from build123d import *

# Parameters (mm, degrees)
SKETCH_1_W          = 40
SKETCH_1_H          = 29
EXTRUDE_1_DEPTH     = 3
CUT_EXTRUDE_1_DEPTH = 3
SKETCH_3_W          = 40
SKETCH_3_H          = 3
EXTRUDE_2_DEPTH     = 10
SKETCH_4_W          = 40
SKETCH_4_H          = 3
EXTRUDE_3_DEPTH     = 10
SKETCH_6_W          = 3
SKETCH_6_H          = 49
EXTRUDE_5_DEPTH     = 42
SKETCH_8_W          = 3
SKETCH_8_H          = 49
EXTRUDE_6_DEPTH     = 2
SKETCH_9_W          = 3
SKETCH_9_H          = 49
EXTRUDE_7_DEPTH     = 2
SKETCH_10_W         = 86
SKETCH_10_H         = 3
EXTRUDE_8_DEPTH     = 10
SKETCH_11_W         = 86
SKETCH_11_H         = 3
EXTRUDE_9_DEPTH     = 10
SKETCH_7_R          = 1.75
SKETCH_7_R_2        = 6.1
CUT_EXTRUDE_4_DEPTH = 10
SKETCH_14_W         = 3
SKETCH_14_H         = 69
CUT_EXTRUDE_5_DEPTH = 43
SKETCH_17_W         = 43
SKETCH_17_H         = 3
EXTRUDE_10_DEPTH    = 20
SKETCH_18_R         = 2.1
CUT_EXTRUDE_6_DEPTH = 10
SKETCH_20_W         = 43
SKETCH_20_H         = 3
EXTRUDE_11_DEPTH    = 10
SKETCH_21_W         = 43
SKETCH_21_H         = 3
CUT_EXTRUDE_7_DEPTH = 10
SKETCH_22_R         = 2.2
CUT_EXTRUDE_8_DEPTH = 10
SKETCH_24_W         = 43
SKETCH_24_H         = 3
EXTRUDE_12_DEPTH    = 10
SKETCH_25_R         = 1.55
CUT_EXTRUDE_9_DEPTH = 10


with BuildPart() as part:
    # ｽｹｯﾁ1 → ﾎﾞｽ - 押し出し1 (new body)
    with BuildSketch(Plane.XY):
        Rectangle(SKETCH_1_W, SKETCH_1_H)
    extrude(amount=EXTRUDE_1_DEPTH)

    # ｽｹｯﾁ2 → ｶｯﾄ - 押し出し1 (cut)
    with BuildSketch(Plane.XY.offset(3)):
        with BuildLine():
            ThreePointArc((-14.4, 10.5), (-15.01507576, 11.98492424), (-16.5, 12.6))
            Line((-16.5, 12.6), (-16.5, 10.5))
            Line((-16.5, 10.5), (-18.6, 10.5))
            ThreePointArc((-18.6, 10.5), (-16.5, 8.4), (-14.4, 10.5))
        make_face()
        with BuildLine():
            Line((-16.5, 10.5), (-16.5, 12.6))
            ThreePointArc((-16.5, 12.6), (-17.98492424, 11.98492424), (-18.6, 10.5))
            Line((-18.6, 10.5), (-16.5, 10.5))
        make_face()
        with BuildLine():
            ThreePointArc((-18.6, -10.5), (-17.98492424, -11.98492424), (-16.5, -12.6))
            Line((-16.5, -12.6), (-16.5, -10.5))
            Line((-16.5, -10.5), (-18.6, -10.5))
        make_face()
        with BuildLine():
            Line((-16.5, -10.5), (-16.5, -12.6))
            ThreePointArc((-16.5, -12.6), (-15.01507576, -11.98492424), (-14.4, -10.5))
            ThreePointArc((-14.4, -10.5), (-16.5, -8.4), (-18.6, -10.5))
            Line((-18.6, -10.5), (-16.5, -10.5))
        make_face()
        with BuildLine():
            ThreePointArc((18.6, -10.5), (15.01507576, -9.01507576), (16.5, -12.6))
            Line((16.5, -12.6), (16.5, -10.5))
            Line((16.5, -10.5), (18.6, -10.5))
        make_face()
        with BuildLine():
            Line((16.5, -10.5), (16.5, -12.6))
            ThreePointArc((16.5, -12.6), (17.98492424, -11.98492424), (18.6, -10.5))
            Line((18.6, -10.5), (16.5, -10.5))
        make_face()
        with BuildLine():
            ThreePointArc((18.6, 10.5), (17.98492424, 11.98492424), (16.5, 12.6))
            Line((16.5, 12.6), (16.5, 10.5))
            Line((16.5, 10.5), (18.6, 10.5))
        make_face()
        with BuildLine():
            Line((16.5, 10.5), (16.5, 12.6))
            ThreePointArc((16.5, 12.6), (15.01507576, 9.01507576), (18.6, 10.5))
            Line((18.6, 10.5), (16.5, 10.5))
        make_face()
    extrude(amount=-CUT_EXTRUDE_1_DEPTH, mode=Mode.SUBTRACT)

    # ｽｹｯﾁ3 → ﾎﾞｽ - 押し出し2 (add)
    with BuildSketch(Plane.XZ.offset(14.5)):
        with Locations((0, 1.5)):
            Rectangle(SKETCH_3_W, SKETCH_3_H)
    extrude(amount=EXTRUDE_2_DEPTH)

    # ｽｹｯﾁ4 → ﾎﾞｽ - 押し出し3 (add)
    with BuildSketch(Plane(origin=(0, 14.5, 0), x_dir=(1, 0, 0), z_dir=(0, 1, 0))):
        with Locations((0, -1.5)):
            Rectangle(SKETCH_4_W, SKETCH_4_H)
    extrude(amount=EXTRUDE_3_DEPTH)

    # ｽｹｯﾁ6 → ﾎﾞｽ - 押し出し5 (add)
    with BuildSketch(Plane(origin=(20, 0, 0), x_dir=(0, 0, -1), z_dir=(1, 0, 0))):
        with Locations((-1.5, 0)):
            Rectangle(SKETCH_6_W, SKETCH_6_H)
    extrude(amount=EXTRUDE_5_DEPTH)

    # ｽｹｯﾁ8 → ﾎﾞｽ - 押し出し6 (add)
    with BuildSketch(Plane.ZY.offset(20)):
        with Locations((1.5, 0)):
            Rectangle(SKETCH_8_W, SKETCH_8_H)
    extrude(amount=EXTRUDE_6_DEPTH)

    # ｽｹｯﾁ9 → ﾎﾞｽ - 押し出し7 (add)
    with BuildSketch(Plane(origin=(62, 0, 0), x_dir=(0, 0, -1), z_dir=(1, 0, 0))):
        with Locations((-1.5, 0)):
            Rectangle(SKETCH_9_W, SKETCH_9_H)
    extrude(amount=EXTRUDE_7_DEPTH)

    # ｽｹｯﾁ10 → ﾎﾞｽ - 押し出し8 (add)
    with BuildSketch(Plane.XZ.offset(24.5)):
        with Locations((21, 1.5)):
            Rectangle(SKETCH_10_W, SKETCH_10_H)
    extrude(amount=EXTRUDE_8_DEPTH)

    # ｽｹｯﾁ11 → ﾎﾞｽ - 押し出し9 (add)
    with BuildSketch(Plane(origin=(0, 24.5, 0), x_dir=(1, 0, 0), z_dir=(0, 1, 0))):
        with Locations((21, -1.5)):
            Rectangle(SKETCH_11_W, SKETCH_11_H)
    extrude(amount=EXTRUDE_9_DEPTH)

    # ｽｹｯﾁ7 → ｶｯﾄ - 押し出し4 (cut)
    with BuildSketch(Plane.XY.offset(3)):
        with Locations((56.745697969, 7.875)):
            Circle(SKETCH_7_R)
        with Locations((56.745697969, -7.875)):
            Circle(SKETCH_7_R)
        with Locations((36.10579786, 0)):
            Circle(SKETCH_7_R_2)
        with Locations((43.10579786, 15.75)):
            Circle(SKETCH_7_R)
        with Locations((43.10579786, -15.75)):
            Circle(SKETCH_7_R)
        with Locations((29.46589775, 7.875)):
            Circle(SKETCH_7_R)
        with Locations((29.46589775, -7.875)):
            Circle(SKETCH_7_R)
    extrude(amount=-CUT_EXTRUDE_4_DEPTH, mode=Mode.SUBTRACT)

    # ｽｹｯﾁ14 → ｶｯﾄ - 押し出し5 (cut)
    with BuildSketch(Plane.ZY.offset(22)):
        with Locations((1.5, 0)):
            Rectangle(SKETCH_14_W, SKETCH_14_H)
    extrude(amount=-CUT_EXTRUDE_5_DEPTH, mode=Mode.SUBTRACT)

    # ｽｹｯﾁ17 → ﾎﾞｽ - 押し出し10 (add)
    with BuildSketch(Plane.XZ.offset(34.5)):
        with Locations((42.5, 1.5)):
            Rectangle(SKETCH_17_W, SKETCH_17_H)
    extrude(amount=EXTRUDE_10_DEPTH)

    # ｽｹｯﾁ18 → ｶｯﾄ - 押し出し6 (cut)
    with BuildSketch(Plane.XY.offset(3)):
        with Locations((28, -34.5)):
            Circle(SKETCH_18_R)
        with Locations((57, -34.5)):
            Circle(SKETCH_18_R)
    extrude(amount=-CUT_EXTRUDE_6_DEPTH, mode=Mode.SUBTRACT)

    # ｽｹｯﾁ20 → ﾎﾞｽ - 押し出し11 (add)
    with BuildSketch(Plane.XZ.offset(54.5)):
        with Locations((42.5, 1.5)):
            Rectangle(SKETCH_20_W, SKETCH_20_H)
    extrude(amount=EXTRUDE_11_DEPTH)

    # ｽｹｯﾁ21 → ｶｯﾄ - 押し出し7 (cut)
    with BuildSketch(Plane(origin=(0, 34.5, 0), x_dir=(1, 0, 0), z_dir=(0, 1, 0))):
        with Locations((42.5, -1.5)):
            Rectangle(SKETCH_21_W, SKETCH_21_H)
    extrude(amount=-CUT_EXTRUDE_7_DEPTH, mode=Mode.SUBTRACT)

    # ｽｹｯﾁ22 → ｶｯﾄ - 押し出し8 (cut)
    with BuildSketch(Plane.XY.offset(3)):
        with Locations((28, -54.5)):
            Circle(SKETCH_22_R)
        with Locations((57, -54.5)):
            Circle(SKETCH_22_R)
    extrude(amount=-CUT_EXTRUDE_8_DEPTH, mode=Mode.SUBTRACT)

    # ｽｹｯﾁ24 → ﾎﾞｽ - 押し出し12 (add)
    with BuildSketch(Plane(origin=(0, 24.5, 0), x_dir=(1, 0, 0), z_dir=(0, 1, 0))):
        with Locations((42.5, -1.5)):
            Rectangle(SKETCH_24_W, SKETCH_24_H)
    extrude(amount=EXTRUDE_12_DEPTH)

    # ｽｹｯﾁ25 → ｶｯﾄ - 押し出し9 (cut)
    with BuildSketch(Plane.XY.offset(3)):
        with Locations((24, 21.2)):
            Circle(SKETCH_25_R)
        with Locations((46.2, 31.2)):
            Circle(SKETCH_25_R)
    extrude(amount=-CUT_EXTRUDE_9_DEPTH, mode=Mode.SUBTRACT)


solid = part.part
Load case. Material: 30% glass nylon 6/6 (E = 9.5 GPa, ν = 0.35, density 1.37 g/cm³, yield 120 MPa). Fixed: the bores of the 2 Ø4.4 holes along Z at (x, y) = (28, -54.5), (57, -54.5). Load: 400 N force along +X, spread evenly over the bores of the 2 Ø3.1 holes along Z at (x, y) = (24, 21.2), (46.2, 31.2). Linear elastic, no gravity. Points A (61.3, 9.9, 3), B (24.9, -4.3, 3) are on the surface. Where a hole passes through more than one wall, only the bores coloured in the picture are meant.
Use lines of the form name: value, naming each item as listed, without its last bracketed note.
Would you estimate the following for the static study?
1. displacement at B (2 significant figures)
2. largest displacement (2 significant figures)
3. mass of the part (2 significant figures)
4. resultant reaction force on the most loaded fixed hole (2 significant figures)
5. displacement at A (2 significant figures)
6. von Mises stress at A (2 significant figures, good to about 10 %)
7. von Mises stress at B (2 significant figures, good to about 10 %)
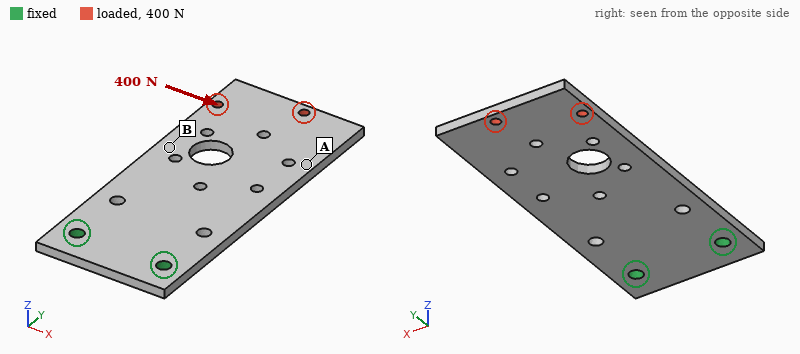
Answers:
displacement at B: 0.29 mm
largest displacement: 0.63 mm
mass of the part: 16 g
resultant reaction force on the most loaded fixed hole: 1.1 kN
displacement at A: 0.41 mm
von Mises stress at A: 5.8 MPa
von Mises stress at B: 16 MPa
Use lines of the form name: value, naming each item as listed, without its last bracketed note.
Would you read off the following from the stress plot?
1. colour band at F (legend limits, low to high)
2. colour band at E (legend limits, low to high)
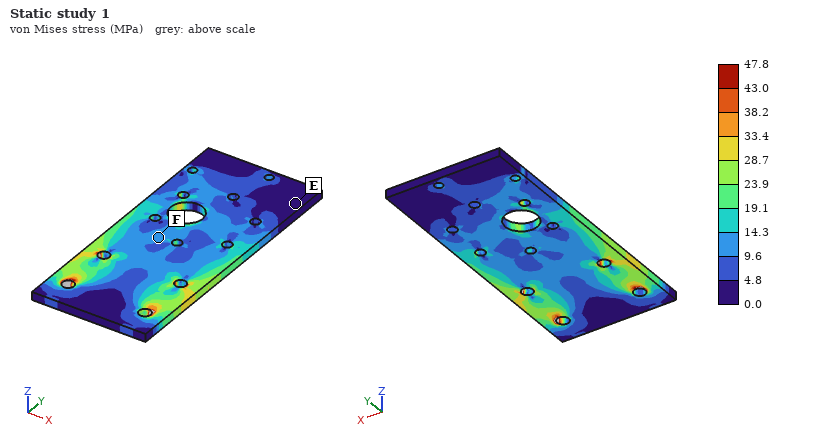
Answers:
colour band at F: 9.6 to 14.3 MPa
colour band at E: 0.0 to 4.8 MPa
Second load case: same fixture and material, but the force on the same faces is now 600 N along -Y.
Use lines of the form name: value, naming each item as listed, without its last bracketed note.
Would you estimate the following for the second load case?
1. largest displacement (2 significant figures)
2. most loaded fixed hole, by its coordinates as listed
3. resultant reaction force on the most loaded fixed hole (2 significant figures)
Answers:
largest displacement: 0.15 mm
most loaded fixed hole, by its coordinates as listed: (28, -54.5)
resultant reaction force on the most loaded fixed hole: 450 N
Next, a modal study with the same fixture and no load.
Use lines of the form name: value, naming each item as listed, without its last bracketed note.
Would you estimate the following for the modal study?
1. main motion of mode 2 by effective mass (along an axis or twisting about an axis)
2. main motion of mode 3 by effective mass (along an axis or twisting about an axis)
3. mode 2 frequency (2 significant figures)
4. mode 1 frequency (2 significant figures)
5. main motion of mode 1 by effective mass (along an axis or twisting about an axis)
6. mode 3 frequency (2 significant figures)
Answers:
main motion of mode 2 by effective mass: twisting about Y
main motion of mode 3 by effective mass: along Z
mode 2 frequency: 690 Hz
mode 1 frequency: 160 Hz
main motion of mode 1 by effective mass: along Z
mode 3 frequency: 980 Hz
